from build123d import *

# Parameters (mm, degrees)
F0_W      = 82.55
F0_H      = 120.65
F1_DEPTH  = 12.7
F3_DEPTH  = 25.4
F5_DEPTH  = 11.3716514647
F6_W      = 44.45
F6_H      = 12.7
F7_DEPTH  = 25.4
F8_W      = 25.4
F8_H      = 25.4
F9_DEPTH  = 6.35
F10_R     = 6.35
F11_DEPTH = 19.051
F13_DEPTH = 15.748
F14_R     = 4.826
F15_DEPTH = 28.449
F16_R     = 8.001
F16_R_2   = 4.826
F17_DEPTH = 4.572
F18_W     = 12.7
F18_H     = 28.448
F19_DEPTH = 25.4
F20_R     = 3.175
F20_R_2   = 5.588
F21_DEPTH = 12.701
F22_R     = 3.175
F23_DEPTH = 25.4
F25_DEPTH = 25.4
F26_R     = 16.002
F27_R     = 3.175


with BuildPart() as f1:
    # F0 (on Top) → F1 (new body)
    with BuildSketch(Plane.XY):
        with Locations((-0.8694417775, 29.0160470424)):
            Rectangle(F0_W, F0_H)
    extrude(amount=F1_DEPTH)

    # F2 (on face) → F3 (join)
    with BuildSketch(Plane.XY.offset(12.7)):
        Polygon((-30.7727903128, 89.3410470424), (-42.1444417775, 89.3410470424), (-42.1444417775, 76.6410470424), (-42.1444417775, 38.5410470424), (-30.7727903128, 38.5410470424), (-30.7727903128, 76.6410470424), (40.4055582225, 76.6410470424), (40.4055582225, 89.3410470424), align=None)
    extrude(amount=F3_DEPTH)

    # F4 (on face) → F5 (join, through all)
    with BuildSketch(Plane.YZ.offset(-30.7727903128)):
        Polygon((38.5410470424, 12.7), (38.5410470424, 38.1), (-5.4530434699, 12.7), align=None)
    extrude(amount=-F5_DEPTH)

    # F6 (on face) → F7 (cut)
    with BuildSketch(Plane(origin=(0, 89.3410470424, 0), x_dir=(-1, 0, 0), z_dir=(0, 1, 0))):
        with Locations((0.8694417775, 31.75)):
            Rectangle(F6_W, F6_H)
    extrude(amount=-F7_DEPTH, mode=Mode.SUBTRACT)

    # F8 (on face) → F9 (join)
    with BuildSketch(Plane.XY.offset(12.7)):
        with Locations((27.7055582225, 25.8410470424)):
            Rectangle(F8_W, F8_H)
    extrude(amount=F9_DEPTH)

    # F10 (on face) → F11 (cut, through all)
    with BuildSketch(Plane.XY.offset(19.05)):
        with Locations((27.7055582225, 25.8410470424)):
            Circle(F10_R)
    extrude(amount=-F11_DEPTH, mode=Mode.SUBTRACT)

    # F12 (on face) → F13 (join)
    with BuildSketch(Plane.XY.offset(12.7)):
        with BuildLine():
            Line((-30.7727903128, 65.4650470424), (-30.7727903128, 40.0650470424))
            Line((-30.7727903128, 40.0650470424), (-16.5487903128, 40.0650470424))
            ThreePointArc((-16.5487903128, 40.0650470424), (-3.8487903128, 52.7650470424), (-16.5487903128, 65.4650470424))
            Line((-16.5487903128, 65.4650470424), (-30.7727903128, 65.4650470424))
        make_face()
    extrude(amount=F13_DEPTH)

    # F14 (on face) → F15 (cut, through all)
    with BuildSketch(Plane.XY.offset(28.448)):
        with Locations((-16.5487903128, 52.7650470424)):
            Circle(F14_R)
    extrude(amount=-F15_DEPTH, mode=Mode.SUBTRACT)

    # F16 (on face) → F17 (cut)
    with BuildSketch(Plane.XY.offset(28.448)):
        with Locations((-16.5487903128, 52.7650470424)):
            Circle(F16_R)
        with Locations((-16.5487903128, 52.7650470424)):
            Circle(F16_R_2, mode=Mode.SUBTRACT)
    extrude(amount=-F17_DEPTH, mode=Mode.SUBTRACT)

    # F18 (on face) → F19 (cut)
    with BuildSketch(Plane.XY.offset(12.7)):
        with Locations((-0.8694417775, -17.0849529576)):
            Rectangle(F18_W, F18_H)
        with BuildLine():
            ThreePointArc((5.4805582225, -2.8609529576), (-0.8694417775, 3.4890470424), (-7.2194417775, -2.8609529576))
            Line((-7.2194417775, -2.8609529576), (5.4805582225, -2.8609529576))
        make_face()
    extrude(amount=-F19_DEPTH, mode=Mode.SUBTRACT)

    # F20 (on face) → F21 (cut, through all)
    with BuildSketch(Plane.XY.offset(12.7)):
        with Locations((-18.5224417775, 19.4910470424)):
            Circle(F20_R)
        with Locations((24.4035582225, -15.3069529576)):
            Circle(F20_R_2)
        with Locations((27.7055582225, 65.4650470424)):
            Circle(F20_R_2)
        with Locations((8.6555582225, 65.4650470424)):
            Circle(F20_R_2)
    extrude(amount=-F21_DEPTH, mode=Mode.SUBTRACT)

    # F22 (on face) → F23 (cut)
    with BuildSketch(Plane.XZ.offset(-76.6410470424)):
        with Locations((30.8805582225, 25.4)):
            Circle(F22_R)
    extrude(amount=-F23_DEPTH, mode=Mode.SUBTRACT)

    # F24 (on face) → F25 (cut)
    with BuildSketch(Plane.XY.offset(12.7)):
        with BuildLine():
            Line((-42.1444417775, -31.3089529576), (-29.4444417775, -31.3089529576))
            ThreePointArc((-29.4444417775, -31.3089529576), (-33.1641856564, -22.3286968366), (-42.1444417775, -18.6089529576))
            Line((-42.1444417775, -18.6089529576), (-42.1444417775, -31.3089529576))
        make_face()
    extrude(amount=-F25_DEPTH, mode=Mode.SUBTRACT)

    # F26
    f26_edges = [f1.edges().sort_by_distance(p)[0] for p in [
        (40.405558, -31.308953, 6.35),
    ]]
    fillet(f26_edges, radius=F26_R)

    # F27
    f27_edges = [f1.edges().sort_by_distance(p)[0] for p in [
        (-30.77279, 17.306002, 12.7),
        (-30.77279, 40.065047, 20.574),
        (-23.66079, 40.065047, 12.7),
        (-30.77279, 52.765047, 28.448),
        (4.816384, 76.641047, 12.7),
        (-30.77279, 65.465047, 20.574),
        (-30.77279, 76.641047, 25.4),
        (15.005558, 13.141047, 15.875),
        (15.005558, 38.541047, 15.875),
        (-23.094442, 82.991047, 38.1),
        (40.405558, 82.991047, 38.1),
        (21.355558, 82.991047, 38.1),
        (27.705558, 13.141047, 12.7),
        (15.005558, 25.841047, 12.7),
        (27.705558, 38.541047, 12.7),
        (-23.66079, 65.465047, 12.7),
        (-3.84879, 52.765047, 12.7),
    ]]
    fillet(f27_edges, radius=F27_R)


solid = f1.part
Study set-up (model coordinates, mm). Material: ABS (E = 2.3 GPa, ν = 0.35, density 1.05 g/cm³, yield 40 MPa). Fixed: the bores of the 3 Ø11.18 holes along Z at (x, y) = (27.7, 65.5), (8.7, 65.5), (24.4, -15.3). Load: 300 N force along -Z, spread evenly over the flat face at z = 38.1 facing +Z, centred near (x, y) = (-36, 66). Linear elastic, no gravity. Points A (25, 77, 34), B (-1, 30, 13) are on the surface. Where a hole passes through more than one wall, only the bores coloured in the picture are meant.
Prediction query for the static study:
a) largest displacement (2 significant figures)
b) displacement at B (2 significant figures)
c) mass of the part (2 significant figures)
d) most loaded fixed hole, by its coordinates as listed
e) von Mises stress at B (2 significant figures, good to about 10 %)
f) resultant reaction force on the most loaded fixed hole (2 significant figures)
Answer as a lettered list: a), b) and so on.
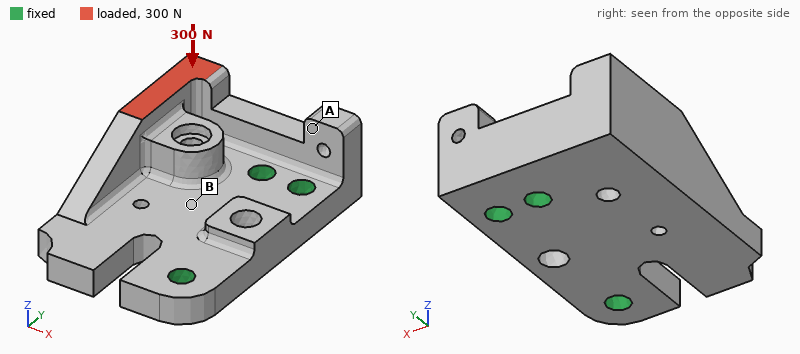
a) 0.30 mm
b) 0.048 mm
c) 170 g
d) (8.7, 65.5)
e) 1.6 MPa
f) 530 N
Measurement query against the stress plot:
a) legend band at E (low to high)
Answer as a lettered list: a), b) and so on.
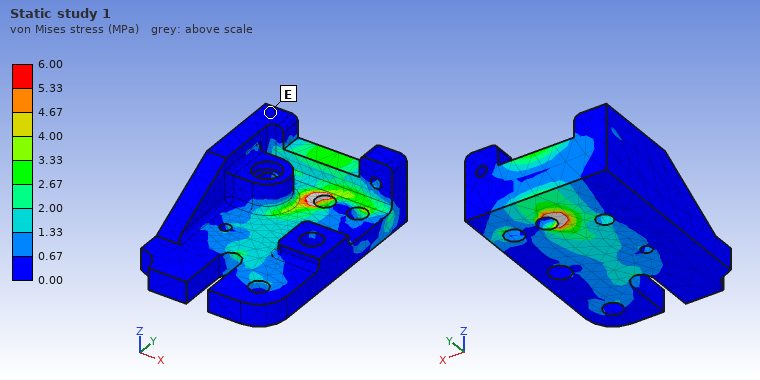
a) 0.00 to 0.67 MPa
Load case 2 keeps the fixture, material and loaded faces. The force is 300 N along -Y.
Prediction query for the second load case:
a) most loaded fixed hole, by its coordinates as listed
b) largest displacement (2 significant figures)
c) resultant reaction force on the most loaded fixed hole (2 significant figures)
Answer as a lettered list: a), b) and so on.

a) (8.7, 65.5)
b) 0.29 mm
c) 320 N
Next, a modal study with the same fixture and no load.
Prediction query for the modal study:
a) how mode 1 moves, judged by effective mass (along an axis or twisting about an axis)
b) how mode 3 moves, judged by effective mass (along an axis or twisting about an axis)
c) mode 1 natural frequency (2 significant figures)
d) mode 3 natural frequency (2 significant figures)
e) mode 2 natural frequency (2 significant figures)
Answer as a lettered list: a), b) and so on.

a) along Z
b) along Y
c) 600 Hz
d) 1600 Hz
e) 1000 Hz
